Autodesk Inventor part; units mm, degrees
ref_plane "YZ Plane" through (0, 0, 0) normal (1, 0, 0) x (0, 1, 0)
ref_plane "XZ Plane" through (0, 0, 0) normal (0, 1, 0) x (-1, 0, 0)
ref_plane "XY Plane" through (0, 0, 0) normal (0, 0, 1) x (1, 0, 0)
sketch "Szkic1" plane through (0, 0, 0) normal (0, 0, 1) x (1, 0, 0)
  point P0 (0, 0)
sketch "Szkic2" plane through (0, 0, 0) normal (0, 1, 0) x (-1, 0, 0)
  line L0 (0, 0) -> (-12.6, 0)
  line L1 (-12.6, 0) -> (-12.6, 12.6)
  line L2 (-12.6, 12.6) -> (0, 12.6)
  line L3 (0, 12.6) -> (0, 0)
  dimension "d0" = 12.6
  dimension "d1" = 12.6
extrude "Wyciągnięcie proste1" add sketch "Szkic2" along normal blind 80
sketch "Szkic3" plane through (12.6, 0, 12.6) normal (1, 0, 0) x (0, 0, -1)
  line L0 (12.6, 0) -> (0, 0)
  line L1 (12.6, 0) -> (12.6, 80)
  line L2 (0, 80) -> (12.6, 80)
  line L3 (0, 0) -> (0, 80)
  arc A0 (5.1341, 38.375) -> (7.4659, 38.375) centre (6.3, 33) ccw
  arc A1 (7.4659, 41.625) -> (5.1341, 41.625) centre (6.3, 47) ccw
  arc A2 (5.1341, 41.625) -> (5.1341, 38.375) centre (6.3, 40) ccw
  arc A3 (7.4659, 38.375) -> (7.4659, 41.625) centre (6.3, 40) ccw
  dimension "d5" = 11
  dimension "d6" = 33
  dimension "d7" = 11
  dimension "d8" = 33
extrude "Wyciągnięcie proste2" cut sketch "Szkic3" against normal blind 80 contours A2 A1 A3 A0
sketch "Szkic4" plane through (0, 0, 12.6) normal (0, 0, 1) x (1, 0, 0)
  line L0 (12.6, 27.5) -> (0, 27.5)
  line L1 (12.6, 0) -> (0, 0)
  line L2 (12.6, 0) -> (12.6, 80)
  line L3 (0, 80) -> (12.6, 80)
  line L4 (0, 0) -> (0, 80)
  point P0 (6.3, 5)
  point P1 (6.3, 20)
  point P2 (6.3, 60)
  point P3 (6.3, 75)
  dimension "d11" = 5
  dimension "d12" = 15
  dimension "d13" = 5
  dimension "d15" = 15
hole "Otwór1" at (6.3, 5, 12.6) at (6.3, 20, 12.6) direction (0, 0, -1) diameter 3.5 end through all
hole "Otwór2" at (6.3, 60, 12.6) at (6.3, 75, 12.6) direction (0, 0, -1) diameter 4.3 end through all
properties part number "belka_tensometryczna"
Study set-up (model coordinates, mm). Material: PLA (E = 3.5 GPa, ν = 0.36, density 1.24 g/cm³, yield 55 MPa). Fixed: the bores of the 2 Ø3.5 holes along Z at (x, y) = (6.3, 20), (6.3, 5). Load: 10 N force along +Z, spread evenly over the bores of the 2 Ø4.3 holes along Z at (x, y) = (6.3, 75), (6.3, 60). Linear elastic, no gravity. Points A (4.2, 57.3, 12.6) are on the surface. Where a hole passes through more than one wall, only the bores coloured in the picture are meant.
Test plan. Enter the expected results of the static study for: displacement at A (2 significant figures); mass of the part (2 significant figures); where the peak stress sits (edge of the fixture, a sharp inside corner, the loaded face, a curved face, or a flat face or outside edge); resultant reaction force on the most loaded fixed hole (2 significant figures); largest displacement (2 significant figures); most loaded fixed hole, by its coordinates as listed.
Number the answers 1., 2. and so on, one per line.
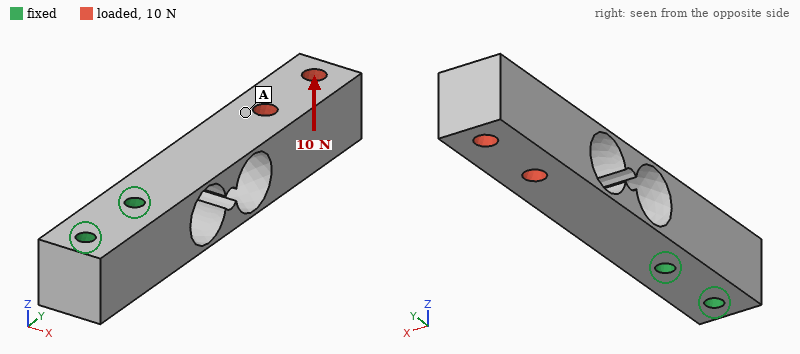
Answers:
1. 0.87 mm
2. 12 g
3. a curved face
4. 15 N
5. 0.93 mm
6. (6.3, 20)
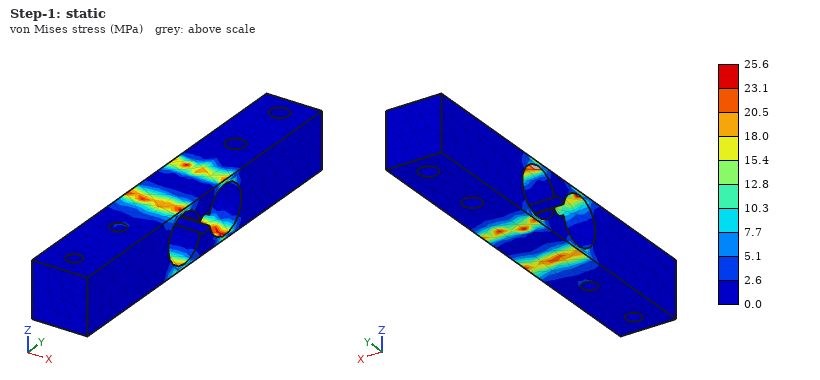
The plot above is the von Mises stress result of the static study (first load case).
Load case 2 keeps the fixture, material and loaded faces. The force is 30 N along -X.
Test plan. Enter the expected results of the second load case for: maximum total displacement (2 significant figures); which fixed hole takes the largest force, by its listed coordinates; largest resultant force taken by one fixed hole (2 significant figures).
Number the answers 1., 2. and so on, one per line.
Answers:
1. 0.89 mm
2. (6.3, 20)
3. 84 N
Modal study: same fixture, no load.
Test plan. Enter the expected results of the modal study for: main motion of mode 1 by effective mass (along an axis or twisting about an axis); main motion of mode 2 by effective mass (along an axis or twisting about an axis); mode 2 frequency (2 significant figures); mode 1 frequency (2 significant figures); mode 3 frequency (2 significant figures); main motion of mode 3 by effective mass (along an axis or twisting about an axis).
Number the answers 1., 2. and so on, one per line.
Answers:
1. along Z
2. along X
3. 490 Hz
4. 230 Hz
5. 1600 Hz
6. twisting about Y
